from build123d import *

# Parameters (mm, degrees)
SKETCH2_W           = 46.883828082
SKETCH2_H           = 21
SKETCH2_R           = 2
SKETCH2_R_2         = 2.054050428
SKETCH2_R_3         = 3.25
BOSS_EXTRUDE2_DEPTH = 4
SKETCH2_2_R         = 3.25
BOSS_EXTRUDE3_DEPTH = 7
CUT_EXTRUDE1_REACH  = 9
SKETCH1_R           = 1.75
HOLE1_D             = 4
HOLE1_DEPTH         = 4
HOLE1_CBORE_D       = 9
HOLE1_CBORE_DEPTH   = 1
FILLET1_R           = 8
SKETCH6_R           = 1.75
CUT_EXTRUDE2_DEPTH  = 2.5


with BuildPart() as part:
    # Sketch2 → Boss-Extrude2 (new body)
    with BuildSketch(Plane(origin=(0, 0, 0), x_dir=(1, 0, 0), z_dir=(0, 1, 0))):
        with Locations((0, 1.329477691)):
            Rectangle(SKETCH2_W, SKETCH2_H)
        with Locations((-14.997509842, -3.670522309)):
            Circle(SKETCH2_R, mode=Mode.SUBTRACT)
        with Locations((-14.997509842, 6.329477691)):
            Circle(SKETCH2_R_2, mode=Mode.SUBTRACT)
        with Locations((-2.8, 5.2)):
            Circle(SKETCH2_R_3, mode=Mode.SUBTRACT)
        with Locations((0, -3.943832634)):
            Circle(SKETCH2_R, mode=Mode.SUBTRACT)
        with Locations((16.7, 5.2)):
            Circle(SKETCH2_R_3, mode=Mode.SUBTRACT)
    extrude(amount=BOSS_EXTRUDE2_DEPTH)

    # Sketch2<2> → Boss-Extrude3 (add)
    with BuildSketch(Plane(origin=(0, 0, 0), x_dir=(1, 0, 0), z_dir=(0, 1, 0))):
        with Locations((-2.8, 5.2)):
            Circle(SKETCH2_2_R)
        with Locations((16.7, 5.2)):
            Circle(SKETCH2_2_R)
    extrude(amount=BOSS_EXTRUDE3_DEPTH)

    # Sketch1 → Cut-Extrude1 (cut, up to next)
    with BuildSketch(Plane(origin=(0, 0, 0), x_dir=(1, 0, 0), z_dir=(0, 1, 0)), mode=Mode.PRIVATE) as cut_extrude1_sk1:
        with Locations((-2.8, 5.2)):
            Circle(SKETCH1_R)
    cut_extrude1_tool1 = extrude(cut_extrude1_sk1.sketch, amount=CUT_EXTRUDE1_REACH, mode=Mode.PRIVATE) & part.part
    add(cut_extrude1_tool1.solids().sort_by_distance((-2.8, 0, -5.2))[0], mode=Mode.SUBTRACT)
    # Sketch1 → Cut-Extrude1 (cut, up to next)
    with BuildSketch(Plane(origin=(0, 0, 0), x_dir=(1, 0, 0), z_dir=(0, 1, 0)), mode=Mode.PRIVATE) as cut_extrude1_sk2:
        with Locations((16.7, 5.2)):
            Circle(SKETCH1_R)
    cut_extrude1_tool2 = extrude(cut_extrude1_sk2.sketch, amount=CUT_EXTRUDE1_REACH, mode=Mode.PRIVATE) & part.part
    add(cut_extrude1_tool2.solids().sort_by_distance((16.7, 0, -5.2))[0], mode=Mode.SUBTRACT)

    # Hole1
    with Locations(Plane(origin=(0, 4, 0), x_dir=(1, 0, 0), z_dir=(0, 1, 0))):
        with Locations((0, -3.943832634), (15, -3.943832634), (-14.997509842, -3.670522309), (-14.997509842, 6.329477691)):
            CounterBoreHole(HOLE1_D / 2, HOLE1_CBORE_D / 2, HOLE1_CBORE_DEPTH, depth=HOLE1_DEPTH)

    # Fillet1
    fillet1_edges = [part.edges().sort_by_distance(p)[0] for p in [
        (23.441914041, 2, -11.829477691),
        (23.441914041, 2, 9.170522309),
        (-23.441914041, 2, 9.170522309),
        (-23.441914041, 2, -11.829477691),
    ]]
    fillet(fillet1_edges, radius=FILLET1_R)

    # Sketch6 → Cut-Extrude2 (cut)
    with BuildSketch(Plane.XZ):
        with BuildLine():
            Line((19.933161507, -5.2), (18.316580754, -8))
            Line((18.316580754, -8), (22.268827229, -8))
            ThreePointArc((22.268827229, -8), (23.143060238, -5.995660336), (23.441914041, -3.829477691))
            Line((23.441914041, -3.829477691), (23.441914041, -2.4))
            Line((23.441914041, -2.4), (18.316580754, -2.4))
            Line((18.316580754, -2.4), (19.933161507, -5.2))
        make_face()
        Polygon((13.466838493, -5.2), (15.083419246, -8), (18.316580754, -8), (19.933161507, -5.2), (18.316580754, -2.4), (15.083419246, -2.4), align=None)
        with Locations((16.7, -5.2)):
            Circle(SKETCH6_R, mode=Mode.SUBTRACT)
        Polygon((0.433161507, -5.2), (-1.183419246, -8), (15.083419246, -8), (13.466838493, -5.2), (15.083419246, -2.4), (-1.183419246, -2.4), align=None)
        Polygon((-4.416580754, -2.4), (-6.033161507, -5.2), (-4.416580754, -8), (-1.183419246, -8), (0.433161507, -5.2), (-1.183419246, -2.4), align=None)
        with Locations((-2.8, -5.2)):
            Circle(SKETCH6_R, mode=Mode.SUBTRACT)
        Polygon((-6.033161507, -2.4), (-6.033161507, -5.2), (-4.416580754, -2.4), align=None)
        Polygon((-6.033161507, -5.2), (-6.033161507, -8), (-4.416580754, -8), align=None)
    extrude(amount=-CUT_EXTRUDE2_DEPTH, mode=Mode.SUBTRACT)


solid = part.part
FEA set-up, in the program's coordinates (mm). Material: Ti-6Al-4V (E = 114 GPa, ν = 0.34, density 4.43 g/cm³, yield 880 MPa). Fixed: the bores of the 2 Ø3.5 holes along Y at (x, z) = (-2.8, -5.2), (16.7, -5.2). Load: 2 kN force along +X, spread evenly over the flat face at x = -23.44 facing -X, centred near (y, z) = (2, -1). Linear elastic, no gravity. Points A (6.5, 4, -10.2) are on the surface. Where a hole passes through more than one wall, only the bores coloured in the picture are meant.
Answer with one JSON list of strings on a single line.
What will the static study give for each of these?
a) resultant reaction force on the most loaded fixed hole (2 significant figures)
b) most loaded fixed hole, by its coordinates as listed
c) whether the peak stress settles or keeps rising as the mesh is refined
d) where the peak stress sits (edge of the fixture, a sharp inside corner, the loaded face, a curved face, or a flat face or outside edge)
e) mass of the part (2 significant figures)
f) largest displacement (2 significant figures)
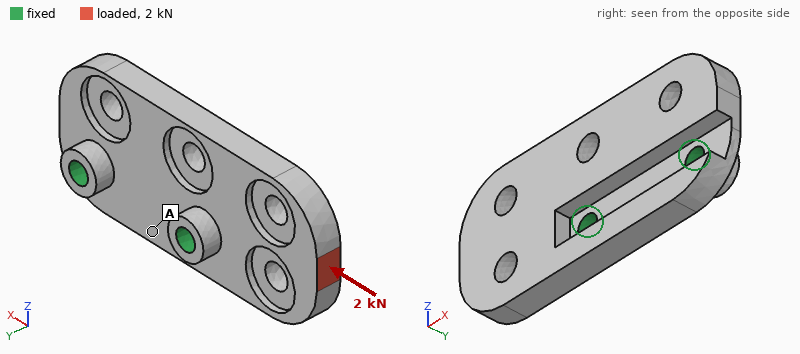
["1.4 kN", "(-2.8, -5.2)", "keeps rising", "edge of the fixture", "13 g", "18 µm"]
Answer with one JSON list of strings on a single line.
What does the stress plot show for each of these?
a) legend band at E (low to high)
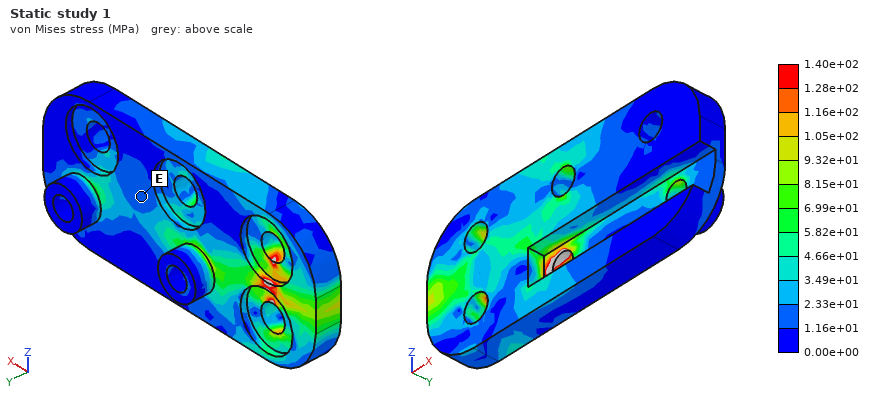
["1.16e+01 to 2.33e+01 MPa"]
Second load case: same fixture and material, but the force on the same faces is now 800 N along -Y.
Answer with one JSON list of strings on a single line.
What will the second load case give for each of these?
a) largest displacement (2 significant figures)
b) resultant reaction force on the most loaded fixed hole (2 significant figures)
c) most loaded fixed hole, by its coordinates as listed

["0.39 mm", "1.7 kN", "(-2.8, -5.2)"]
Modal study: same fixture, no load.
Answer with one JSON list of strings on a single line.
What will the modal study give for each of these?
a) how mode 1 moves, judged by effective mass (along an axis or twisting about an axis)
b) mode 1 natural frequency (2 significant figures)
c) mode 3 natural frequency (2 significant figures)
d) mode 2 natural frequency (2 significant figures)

["along Y", "6000 Hz", "13 kHz", "7800 Hz"]
